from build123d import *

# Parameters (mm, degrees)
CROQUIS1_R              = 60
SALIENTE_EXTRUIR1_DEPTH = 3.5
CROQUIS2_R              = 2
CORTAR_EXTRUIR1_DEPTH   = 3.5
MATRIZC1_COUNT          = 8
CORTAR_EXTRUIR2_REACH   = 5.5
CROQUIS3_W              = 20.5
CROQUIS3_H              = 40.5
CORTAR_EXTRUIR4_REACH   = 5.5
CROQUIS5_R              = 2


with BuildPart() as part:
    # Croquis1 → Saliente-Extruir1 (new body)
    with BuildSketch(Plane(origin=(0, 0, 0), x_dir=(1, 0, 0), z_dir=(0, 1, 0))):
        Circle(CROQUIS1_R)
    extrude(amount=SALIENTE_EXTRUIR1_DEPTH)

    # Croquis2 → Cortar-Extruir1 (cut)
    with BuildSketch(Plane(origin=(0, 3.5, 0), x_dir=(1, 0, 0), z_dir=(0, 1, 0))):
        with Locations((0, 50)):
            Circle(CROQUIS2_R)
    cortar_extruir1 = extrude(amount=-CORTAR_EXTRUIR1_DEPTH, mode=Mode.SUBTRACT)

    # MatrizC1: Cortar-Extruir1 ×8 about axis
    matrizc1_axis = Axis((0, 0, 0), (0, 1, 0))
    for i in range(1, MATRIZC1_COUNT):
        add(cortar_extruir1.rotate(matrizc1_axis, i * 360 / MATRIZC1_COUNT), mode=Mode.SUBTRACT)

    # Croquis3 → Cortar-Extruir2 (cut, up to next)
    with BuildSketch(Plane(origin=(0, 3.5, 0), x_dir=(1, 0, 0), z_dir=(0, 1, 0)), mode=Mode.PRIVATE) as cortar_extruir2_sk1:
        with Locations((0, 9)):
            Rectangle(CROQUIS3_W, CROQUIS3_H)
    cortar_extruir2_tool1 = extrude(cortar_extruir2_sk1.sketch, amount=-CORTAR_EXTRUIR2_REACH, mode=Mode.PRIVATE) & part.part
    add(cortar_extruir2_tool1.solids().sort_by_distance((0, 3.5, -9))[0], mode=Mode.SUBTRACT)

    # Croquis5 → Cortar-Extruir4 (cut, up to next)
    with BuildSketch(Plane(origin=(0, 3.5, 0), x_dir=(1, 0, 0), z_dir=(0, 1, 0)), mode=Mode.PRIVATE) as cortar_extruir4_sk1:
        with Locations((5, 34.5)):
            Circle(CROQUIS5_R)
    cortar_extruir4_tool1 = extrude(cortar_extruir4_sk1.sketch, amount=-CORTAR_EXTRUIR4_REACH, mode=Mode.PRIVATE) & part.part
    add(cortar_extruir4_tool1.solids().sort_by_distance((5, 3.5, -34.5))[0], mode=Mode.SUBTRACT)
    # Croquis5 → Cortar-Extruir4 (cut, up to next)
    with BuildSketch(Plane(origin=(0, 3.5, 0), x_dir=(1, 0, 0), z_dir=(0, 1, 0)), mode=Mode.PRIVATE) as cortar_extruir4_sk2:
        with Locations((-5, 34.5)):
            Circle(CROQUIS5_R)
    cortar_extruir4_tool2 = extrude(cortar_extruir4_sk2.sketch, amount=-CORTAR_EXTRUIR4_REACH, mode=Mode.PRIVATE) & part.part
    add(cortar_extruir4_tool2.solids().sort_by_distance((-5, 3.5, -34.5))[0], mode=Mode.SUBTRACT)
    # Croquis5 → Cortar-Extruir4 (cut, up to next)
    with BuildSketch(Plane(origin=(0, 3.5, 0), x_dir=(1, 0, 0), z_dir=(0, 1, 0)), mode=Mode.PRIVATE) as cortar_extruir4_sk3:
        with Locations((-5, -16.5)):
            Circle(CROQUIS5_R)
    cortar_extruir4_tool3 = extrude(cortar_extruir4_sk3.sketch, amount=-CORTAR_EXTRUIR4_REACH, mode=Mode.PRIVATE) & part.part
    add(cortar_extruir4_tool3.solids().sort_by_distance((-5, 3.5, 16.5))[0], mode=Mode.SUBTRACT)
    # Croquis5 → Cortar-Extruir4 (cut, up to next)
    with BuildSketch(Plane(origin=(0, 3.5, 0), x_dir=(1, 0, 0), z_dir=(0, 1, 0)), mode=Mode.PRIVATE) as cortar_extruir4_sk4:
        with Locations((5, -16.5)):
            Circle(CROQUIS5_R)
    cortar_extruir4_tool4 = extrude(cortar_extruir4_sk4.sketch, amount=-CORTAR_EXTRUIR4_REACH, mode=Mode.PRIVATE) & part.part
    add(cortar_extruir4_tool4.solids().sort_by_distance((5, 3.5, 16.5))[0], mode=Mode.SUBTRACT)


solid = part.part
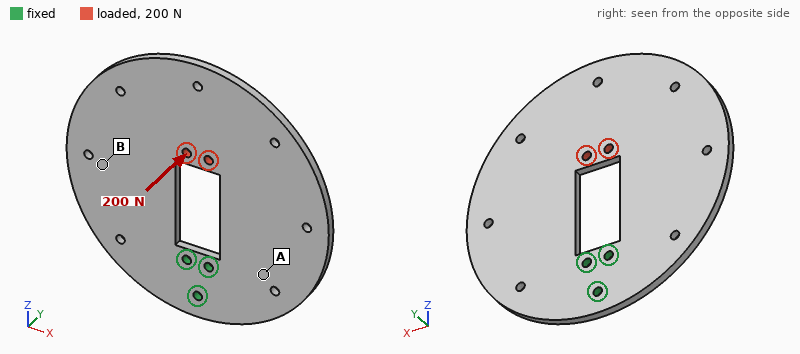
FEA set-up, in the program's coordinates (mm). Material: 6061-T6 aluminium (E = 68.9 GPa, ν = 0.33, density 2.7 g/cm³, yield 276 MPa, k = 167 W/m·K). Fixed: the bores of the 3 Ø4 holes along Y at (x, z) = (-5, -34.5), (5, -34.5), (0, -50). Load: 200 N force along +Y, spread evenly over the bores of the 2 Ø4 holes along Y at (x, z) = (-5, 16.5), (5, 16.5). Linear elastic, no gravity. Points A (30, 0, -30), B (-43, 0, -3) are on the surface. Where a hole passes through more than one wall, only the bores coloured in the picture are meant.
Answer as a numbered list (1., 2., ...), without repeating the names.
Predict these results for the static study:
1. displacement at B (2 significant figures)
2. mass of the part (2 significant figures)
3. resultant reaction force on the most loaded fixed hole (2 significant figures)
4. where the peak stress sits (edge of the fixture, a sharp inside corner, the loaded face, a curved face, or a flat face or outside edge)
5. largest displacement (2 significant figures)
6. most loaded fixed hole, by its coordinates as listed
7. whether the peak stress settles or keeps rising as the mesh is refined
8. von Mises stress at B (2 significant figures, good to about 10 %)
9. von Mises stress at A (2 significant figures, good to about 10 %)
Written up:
1. 0.47 mm
2. 98 g
3. 370 N
4. edge of the fixture
5. 1.7 mm
6. (0, -50)
7. keeps rising
8. 20 MPa
9. 48 MPa
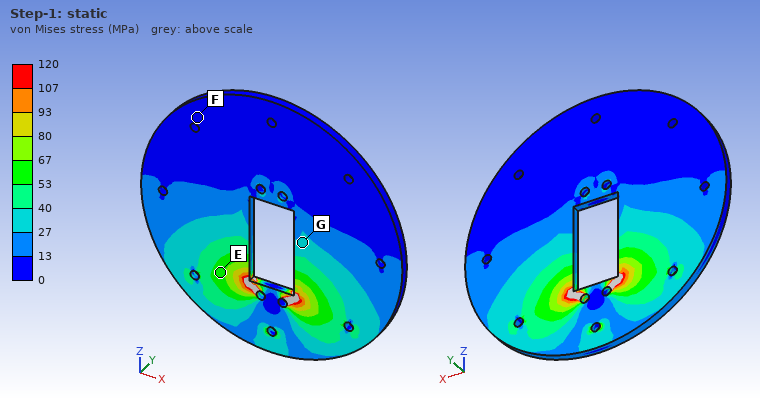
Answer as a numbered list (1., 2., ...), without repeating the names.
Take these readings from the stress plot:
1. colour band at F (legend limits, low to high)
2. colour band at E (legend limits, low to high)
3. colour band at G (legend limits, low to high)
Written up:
1. 0 to 13 MPa
2. 53 to 67 MPa
3. 27 to 40 MPa
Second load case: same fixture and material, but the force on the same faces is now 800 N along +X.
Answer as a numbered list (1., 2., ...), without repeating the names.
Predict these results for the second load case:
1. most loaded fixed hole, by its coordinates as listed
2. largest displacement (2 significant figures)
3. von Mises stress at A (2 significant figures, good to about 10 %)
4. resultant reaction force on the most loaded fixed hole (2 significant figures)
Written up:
1. (0, -50)
2. 0.11 mm
3. 13 MPa
4. 2.0 kN
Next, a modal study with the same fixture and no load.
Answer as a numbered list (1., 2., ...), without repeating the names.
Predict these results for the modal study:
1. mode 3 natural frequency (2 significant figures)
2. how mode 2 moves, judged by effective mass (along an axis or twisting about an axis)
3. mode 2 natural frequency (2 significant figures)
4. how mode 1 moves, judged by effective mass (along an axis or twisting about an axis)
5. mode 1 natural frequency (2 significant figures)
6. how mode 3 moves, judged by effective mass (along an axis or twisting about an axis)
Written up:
1. 1000 Hz
2. twisting about Z
3. 460 Hz
4. along Y
5. 260 Hz
6. along Y
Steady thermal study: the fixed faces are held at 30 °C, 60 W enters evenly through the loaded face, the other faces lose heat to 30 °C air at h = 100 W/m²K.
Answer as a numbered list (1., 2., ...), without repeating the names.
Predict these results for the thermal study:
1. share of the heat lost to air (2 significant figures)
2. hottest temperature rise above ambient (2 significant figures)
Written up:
1. 78 %
2. 74 K
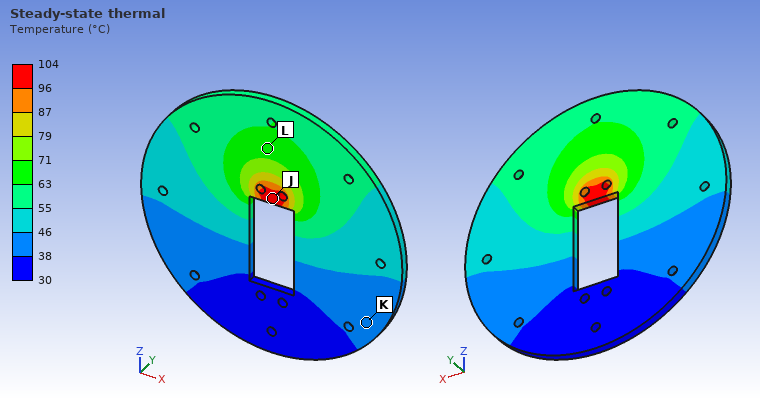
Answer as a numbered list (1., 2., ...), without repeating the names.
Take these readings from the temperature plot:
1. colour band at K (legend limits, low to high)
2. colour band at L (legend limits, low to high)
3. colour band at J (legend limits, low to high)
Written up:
1. 38 to 46 °C
2. 63 to 71 °C
3. 96 to 104 °C
